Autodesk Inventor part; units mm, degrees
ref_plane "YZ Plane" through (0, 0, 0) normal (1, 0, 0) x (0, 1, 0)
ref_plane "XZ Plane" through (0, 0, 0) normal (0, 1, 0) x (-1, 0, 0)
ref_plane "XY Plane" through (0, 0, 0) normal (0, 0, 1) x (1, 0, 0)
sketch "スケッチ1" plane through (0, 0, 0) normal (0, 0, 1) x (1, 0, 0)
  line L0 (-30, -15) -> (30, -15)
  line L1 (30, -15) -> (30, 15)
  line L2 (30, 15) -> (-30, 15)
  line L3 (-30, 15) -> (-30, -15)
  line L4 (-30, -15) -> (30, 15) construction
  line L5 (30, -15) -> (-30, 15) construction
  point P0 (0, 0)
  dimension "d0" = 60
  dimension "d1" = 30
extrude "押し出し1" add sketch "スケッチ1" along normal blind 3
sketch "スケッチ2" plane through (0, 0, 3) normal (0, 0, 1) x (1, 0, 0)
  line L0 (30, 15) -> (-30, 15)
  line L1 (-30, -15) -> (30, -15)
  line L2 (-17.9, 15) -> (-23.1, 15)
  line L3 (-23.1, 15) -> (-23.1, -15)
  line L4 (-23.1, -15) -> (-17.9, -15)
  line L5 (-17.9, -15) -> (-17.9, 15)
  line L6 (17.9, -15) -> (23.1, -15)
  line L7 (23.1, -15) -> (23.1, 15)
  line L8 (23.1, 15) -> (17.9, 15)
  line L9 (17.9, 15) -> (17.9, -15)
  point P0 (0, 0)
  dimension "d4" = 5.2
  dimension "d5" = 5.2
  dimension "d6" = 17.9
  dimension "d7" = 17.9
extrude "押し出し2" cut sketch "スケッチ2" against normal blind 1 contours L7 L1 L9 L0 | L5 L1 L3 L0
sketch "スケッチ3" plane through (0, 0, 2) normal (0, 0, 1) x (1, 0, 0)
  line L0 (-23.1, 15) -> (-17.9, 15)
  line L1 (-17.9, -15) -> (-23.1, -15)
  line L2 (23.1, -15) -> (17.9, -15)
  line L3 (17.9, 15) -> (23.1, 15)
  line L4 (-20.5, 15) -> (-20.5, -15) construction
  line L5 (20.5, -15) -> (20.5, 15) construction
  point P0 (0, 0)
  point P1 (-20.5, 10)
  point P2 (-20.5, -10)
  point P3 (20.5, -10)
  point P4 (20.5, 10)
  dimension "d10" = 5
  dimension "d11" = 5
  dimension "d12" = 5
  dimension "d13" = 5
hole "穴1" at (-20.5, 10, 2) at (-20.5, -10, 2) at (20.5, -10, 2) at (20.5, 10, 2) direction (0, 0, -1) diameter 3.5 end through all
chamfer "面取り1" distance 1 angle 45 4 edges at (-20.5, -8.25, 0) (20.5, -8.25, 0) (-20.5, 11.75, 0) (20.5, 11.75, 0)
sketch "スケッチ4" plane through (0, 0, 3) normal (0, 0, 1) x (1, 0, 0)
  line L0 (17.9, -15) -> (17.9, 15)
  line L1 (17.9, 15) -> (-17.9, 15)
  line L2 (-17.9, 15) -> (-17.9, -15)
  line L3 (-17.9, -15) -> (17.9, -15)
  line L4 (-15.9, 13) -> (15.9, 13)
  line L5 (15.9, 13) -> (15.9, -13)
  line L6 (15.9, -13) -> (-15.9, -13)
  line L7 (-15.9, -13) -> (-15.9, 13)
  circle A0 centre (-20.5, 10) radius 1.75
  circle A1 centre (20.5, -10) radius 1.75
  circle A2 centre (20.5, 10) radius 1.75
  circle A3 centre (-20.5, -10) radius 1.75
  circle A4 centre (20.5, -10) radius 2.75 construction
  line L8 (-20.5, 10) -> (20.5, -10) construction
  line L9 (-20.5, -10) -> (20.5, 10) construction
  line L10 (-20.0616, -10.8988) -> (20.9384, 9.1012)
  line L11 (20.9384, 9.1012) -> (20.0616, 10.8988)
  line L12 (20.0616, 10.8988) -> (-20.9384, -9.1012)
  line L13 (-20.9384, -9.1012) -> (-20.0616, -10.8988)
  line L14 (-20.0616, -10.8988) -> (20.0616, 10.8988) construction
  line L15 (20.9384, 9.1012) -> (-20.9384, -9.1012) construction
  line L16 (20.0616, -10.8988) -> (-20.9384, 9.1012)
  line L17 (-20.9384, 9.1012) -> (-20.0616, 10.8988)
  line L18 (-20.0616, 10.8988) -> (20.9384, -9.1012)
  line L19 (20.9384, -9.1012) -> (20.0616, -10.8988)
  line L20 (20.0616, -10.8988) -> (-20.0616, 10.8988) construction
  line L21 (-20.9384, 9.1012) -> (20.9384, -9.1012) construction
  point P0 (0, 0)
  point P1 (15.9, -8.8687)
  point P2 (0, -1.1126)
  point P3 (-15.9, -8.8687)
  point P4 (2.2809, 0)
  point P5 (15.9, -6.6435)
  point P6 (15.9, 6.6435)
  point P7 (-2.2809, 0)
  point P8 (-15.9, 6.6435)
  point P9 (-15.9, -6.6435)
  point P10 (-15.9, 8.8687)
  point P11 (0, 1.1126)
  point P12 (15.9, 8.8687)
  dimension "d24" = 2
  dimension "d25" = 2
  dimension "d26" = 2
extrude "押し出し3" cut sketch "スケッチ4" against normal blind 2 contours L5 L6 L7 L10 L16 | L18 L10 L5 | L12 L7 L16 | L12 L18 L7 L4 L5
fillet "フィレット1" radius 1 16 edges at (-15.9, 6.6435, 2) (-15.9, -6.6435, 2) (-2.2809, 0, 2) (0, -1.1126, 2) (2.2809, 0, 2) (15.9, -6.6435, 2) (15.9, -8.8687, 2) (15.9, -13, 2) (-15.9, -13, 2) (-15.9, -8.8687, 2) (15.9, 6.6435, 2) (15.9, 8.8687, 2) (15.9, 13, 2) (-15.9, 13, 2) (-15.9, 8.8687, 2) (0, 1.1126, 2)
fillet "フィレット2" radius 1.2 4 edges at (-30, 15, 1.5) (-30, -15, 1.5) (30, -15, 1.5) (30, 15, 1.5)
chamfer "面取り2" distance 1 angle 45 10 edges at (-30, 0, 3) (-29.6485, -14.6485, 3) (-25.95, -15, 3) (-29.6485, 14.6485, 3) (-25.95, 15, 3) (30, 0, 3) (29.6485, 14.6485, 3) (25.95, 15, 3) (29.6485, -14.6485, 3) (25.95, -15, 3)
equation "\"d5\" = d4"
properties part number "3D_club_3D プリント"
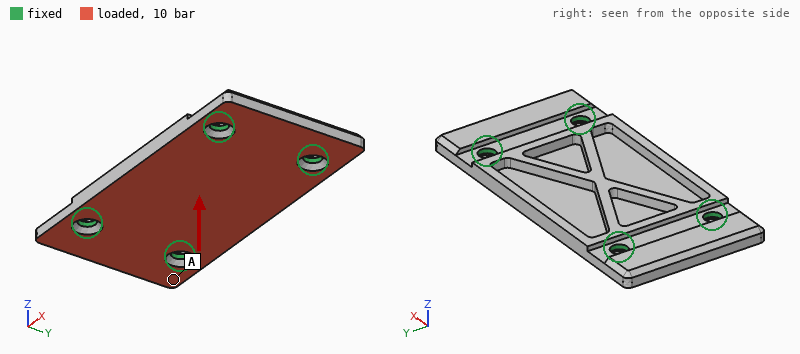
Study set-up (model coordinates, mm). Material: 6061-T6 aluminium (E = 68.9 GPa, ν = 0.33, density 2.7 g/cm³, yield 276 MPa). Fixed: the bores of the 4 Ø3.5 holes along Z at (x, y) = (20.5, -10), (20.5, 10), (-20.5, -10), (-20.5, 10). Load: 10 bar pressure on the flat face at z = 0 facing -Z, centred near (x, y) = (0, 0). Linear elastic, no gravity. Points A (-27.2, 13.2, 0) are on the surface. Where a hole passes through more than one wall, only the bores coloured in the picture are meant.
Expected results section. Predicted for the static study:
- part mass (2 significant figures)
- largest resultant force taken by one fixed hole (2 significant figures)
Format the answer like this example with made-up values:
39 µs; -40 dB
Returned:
9.6 g; 480 N
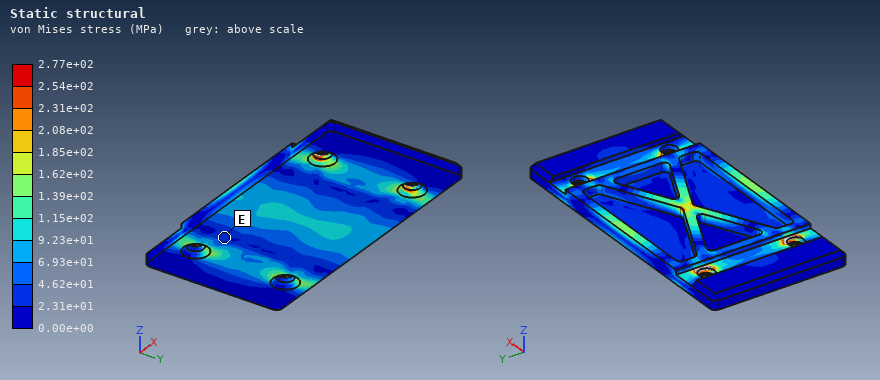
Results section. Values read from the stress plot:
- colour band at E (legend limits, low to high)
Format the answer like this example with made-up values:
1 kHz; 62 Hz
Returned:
2.31e+01 to 4.62e+01 MPa
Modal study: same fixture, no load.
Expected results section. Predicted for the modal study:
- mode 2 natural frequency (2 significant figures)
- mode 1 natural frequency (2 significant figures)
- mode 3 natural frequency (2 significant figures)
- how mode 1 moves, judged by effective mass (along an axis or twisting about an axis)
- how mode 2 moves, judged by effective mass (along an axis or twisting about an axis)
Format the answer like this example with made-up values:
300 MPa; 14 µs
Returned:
8700 Hz; 6800 Hz; 12 kHz; along Z; twisting about X
